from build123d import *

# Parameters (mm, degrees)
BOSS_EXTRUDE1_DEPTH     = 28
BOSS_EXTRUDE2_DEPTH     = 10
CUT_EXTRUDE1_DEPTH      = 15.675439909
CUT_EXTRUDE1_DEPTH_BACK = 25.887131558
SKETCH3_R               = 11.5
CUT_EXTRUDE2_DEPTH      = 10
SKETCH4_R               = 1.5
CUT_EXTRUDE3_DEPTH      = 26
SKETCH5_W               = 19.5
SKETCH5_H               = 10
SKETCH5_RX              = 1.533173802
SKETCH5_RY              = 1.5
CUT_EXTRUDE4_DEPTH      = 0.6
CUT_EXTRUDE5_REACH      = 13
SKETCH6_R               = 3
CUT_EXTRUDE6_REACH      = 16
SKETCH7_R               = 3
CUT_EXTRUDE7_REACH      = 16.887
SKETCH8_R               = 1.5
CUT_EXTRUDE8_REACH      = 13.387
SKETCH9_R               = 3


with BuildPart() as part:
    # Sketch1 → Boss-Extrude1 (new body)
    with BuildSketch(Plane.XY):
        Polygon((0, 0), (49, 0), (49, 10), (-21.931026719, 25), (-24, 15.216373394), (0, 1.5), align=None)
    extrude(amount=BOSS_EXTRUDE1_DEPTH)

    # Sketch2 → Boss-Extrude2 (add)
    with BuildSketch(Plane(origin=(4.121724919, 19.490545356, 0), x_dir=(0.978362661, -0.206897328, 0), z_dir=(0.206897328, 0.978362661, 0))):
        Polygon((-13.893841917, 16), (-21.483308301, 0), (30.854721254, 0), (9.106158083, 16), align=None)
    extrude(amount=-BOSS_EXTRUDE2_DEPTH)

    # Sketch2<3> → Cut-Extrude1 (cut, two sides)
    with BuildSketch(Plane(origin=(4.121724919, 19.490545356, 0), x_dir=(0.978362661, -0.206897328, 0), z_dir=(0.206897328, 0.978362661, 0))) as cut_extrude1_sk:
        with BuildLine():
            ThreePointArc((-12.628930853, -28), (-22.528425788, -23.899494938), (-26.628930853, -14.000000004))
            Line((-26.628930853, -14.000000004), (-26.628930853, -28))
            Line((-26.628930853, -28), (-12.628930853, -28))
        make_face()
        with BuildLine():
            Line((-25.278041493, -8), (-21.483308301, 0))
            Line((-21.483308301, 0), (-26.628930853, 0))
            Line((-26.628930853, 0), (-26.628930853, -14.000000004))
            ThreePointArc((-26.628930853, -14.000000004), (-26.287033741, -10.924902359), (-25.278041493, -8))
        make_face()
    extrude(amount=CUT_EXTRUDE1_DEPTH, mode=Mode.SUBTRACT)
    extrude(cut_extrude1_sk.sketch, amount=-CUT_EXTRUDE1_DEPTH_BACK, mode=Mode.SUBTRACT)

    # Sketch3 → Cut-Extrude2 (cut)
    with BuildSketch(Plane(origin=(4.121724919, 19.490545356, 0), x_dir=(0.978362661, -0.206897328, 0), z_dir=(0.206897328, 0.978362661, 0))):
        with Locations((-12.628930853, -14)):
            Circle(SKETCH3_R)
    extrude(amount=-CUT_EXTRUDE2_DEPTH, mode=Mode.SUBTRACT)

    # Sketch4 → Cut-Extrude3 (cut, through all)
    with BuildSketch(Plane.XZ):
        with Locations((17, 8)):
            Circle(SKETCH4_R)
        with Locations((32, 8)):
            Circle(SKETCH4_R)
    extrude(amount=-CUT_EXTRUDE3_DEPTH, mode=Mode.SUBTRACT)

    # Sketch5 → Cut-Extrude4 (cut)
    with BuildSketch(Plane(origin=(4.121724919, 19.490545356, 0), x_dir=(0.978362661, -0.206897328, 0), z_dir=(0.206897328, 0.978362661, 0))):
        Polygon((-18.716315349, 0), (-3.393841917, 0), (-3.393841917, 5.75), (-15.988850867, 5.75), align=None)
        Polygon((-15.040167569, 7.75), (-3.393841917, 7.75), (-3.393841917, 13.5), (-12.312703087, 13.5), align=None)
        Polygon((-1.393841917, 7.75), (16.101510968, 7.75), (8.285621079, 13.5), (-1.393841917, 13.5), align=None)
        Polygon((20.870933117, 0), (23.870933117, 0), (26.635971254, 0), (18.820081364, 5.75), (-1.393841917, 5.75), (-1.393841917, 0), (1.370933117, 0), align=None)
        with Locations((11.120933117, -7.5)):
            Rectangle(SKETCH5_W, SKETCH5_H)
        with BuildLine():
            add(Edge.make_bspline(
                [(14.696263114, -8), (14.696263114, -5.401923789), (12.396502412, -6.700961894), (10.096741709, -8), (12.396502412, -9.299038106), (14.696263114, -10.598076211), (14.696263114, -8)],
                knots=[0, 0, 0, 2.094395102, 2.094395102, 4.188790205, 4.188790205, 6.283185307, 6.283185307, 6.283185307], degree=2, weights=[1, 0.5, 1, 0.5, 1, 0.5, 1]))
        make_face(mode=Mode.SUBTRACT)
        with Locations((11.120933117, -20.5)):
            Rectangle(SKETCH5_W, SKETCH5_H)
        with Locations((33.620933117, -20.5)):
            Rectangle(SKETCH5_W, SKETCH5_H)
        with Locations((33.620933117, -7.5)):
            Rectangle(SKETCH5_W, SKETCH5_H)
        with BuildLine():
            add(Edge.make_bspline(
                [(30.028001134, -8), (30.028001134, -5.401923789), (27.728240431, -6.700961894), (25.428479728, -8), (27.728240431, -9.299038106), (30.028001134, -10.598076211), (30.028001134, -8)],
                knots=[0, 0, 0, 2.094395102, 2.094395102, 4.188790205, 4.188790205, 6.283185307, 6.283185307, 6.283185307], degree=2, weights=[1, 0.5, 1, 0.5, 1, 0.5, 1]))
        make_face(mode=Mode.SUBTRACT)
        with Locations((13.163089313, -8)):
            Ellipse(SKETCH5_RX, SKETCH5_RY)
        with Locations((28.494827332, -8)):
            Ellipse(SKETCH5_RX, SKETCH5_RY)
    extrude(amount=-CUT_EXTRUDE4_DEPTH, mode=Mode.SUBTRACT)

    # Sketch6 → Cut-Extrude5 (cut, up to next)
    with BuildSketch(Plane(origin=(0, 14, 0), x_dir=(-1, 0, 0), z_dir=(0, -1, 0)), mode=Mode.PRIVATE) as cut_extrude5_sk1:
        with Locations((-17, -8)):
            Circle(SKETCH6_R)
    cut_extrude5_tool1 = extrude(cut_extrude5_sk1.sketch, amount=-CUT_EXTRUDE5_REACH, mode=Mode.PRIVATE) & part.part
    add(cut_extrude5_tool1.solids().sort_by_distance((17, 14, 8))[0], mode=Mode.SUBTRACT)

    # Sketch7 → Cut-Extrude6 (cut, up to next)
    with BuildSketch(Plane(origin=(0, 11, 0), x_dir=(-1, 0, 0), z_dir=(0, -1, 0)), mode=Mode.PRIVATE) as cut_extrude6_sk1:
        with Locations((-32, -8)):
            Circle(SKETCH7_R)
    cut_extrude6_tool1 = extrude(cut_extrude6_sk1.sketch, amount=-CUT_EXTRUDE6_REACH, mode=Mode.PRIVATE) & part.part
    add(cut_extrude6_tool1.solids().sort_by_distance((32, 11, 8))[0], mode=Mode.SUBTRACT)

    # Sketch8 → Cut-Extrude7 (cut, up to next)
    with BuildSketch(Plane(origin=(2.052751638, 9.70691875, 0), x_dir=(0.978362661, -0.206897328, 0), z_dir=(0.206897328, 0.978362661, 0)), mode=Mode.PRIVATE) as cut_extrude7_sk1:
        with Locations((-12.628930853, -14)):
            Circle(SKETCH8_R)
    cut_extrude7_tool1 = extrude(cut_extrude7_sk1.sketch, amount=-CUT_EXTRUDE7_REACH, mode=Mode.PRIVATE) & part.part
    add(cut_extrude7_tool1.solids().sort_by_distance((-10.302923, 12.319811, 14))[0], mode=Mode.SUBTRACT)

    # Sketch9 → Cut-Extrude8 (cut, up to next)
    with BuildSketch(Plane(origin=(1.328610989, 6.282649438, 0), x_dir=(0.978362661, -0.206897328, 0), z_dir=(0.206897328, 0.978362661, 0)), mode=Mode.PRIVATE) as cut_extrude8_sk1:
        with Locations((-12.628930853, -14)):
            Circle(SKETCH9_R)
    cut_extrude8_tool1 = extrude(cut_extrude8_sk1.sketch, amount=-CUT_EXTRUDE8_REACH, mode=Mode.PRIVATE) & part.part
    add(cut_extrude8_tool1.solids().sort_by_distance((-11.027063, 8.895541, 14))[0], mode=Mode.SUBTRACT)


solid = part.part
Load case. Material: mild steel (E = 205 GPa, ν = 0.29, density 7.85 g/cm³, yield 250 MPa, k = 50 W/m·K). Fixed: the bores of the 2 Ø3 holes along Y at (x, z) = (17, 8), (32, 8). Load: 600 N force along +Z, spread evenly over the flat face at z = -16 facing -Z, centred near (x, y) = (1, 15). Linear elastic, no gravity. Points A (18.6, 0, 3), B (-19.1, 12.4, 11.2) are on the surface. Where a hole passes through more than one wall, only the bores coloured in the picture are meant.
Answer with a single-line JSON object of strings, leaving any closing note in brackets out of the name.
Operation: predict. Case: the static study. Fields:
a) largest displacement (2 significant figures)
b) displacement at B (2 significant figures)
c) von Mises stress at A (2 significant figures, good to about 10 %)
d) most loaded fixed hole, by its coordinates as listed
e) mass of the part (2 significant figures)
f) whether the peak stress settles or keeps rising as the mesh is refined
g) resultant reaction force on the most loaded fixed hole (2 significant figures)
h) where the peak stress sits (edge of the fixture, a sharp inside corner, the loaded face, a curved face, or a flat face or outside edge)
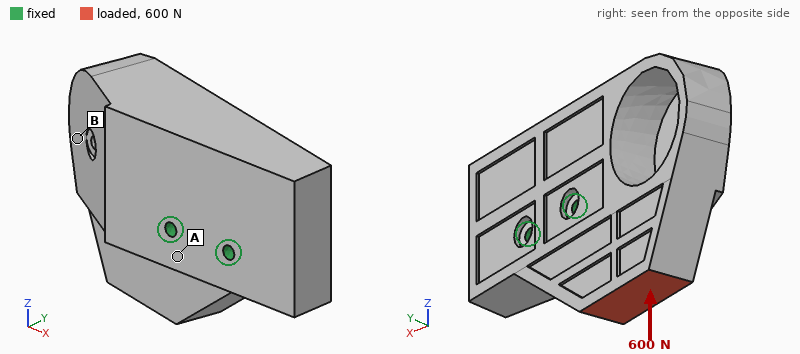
{"largest displacement": "3.0 µm", "displacement at B": "2.0 µm", "von Mises stress at A": "3.4 MPa", "most loaded fixed hole, by its coordinates as listed": "(17, 8)", "mass of the part": "240 g", "whether the peak stress settles or keeps rising as the mesh is refined": "keeps rising", "resultant reaction force on the most loaded fixed hole": "1.1 kN", "where the peak stress sits": "edge of the fixture"}
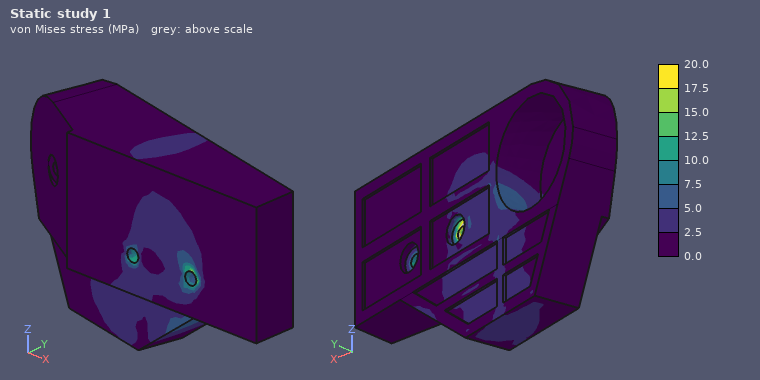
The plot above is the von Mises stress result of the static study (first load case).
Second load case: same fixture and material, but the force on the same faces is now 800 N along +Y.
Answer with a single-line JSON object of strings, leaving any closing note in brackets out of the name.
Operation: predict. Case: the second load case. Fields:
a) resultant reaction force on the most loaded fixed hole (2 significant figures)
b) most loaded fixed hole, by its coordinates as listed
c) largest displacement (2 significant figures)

{"resultant reaction force on the most loaded fixed hole": "1.1 kN", "most loaded fixed hole, by its coordinates as listed": "(17, 8)", "largest displacement": "15 µm"}
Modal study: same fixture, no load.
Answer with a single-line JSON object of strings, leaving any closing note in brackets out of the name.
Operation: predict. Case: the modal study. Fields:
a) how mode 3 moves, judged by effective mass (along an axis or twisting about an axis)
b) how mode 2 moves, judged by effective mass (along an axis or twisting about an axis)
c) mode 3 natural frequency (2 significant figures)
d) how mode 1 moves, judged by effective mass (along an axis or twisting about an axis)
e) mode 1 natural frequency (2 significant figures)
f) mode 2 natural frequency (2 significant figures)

{"how mode 3 moves, judged by effective mass": "twisting about X", "how mode 2 moves, judged by effective mass": "along Z", "mode 3 natural frequency": "9600 Hz", "how mode 1 moves, judged by effective mass": "along Y", "mode 1 natural frequency": "7300 Hz", "mode 2 natural frequency": "8100 Hz"}
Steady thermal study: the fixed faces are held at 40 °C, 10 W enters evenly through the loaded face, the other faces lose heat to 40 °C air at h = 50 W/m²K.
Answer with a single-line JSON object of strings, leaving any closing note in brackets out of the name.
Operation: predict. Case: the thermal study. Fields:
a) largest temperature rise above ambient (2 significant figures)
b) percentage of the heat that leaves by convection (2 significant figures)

{"largest temperature rise above ambient": "20 K", "percentage of the heat that leaves by convection": "20 %"}
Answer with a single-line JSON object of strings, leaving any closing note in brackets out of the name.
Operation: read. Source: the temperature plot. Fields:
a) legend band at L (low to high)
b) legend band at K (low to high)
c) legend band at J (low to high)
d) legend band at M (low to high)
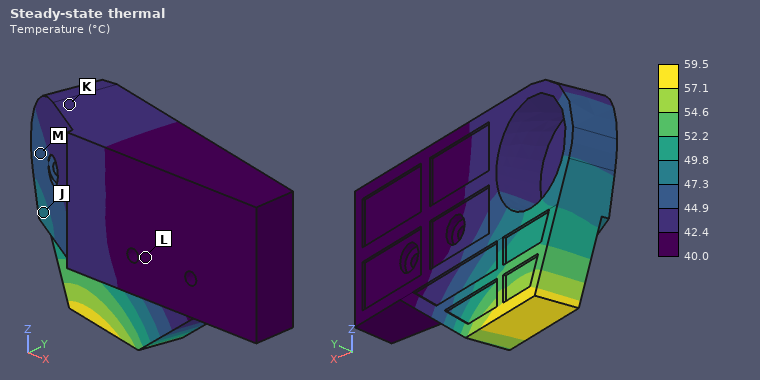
{"legend band at L": "40.0 to 42.4 °C", "legend band at K": "42.4 to 44.9 °C", "legend band at J": "47.3 to 49.8 °C", "legend band at M": "44.9 to 47.3 °C"}
